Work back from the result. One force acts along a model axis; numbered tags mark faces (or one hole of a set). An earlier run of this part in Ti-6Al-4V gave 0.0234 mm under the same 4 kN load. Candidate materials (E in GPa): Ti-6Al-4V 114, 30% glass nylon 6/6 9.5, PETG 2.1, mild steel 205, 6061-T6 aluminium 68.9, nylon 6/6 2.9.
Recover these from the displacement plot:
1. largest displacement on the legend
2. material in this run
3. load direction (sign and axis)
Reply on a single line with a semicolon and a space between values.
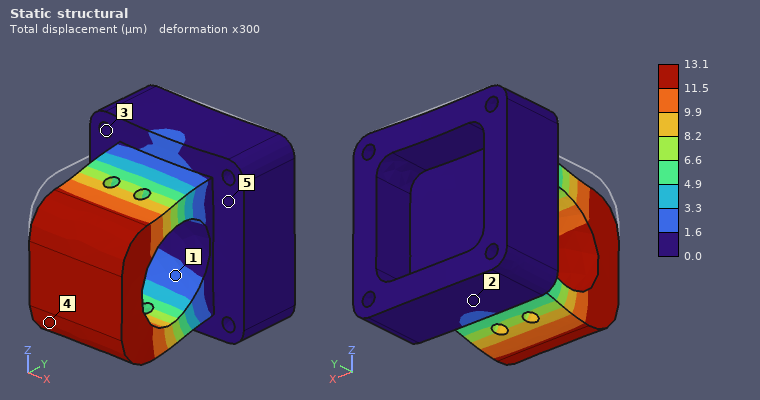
13.1 µm; mild steel; -Z
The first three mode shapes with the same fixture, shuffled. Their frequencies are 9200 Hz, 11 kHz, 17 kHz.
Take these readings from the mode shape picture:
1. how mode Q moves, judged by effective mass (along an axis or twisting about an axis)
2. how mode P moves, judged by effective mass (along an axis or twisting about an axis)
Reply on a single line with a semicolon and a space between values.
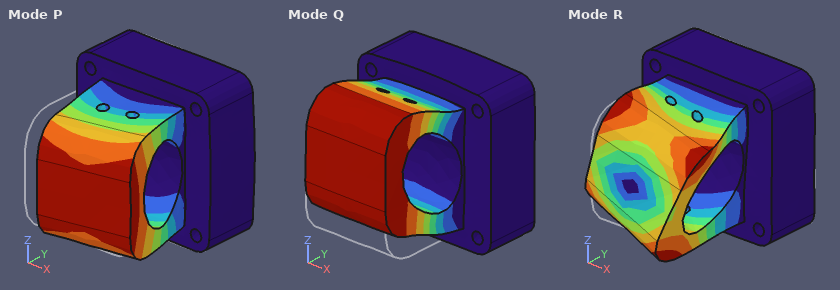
along Z; along X
